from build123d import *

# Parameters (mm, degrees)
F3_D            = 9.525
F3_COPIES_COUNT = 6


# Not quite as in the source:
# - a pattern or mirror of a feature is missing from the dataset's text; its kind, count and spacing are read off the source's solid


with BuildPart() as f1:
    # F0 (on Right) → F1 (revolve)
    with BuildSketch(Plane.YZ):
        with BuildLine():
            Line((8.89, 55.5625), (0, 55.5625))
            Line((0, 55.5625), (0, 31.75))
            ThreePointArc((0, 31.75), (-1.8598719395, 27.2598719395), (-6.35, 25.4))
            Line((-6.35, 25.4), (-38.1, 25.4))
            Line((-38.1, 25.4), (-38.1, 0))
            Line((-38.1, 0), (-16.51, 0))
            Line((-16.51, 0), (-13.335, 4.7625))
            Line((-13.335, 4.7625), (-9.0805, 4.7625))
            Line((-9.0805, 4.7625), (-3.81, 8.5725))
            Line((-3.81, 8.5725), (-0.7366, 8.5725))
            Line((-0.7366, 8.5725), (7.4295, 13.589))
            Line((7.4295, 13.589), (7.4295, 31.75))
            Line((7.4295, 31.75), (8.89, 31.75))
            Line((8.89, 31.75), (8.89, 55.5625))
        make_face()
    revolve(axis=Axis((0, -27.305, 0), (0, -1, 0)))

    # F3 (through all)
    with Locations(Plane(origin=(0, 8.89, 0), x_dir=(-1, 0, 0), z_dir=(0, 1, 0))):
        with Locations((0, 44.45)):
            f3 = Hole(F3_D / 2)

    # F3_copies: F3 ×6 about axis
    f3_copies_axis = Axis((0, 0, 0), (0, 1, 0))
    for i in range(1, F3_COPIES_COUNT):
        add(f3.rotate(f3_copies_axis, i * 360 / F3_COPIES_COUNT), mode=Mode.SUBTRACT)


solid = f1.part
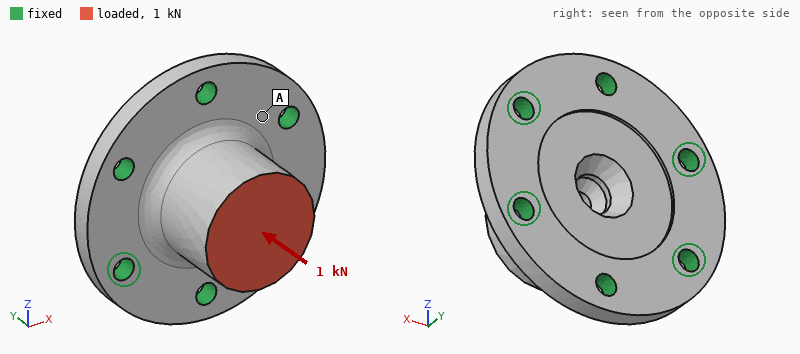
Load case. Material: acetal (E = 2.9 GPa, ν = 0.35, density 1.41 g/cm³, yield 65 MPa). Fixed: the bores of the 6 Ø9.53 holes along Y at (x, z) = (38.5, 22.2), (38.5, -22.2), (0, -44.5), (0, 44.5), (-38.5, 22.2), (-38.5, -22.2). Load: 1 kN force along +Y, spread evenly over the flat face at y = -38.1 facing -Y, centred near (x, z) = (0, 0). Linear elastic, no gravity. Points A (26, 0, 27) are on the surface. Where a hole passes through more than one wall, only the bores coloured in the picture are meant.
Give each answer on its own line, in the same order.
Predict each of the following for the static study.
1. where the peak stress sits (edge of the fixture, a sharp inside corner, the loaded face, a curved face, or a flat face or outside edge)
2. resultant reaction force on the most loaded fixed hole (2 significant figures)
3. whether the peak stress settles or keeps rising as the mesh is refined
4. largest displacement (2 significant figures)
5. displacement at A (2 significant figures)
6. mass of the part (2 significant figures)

edge of the fixture
210 N
keeps rising
41 µm
12 µm
210 g
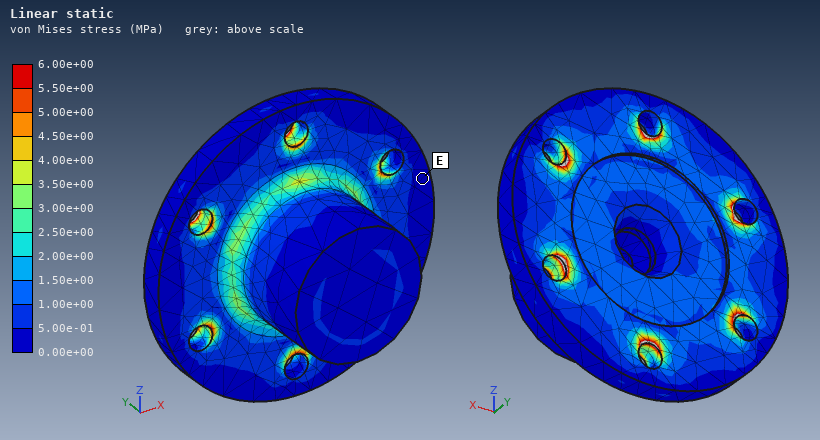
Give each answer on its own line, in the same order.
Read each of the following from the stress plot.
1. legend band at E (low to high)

0.00e+00 to 5.00e-01 MPa
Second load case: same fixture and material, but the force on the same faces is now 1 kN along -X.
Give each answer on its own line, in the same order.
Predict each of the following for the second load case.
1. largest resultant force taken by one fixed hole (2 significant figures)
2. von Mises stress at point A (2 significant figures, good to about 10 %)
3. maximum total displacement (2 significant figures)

430 N
1.4 MPa
0.15 mm
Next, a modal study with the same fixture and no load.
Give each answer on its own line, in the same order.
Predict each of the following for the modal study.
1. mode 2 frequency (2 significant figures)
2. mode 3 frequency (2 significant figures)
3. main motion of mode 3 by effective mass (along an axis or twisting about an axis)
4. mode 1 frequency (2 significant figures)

2000 Hz
2300 Hz
along Y
2000 Hz
